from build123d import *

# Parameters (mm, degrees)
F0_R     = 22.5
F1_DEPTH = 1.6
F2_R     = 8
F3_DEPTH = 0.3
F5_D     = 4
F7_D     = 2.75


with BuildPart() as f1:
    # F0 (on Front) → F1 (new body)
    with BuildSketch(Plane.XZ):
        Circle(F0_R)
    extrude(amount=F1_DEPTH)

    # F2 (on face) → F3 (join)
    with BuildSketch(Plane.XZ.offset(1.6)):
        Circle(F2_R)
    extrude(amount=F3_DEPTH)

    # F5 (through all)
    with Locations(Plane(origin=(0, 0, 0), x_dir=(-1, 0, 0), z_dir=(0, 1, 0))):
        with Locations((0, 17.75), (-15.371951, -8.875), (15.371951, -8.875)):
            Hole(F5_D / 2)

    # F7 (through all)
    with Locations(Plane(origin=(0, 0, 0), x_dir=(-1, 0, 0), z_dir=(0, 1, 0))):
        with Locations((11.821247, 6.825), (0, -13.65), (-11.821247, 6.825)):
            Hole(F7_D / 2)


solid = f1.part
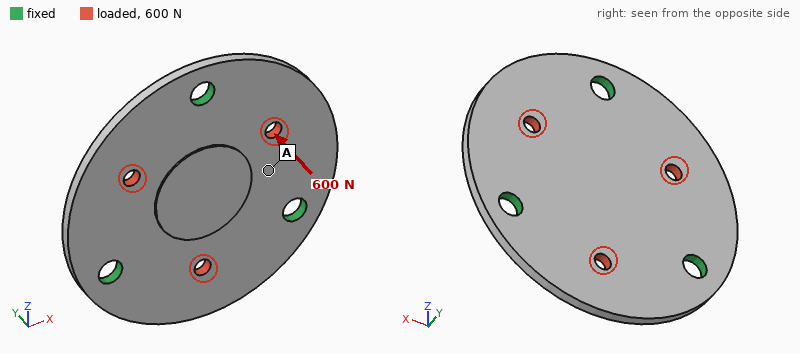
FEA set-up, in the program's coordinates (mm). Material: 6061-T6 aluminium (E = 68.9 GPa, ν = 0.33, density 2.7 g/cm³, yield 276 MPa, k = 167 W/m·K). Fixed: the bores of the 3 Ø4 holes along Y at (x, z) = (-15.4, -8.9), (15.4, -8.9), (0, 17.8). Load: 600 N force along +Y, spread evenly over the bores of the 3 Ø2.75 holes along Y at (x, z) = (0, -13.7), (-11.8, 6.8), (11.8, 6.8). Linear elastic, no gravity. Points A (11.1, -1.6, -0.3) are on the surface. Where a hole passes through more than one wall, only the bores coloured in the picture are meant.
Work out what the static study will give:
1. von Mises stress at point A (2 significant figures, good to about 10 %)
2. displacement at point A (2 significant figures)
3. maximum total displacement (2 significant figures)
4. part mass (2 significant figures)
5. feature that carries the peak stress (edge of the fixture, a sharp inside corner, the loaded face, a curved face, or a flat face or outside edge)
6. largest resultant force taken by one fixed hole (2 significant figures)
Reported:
51 MPa
0.042 mm
0.11 mm
6.8 g
the loaded face
200 N
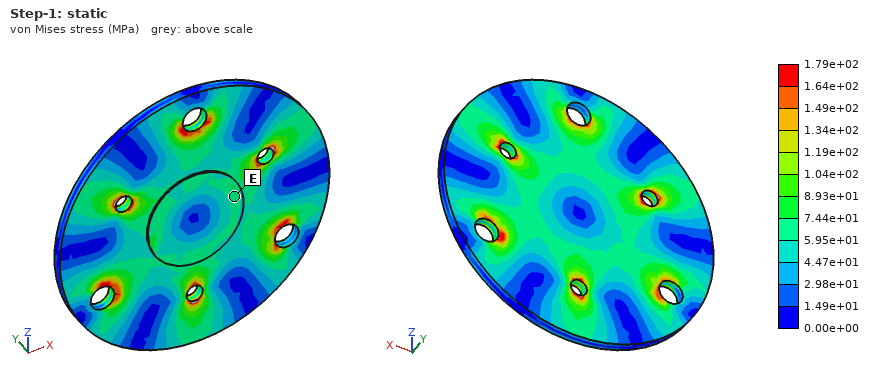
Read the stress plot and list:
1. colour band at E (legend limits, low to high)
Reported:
5.95e+01 to 7.44e+01 MPa
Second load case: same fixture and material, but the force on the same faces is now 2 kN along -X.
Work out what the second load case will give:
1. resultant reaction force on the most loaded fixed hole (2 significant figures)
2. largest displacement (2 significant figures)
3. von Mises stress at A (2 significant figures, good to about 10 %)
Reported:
710 N
9.5 µm
15 MPa
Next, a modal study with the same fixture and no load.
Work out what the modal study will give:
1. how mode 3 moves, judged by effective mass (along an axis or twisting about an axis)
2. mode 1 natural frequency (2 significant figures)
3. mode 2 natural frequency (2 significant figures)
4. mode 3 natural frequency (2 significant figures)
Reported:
along Y
6500 Hz
6500 Hz
7000 Hz
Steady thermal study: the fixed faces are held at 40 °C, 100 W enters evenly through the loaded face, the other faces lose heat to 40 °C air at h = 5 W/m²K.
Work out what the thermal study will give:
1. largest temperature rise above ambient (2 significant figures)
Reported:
87 K
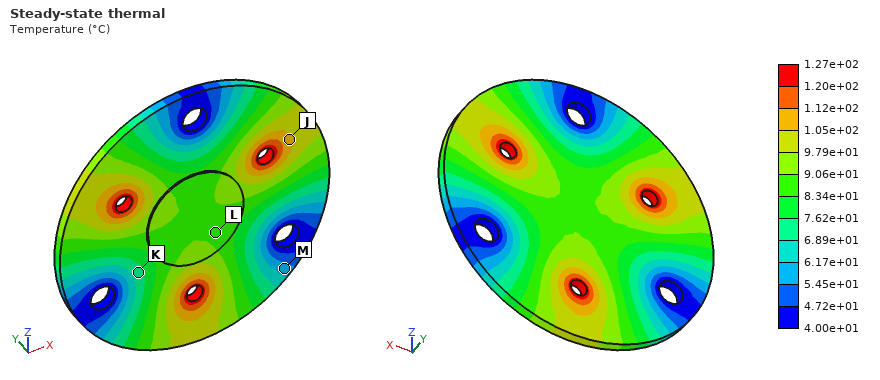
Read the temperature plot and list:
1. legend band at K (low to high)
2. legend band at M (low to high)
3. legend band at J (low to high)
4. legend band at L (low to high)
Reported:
6.89e+01 to 7.62e+01 °C
5.45e+01 to 6.17e+01 °C
1.05e+02 to 1.12e+02 °C
8.34e+01 to 9.06e+01 °C
